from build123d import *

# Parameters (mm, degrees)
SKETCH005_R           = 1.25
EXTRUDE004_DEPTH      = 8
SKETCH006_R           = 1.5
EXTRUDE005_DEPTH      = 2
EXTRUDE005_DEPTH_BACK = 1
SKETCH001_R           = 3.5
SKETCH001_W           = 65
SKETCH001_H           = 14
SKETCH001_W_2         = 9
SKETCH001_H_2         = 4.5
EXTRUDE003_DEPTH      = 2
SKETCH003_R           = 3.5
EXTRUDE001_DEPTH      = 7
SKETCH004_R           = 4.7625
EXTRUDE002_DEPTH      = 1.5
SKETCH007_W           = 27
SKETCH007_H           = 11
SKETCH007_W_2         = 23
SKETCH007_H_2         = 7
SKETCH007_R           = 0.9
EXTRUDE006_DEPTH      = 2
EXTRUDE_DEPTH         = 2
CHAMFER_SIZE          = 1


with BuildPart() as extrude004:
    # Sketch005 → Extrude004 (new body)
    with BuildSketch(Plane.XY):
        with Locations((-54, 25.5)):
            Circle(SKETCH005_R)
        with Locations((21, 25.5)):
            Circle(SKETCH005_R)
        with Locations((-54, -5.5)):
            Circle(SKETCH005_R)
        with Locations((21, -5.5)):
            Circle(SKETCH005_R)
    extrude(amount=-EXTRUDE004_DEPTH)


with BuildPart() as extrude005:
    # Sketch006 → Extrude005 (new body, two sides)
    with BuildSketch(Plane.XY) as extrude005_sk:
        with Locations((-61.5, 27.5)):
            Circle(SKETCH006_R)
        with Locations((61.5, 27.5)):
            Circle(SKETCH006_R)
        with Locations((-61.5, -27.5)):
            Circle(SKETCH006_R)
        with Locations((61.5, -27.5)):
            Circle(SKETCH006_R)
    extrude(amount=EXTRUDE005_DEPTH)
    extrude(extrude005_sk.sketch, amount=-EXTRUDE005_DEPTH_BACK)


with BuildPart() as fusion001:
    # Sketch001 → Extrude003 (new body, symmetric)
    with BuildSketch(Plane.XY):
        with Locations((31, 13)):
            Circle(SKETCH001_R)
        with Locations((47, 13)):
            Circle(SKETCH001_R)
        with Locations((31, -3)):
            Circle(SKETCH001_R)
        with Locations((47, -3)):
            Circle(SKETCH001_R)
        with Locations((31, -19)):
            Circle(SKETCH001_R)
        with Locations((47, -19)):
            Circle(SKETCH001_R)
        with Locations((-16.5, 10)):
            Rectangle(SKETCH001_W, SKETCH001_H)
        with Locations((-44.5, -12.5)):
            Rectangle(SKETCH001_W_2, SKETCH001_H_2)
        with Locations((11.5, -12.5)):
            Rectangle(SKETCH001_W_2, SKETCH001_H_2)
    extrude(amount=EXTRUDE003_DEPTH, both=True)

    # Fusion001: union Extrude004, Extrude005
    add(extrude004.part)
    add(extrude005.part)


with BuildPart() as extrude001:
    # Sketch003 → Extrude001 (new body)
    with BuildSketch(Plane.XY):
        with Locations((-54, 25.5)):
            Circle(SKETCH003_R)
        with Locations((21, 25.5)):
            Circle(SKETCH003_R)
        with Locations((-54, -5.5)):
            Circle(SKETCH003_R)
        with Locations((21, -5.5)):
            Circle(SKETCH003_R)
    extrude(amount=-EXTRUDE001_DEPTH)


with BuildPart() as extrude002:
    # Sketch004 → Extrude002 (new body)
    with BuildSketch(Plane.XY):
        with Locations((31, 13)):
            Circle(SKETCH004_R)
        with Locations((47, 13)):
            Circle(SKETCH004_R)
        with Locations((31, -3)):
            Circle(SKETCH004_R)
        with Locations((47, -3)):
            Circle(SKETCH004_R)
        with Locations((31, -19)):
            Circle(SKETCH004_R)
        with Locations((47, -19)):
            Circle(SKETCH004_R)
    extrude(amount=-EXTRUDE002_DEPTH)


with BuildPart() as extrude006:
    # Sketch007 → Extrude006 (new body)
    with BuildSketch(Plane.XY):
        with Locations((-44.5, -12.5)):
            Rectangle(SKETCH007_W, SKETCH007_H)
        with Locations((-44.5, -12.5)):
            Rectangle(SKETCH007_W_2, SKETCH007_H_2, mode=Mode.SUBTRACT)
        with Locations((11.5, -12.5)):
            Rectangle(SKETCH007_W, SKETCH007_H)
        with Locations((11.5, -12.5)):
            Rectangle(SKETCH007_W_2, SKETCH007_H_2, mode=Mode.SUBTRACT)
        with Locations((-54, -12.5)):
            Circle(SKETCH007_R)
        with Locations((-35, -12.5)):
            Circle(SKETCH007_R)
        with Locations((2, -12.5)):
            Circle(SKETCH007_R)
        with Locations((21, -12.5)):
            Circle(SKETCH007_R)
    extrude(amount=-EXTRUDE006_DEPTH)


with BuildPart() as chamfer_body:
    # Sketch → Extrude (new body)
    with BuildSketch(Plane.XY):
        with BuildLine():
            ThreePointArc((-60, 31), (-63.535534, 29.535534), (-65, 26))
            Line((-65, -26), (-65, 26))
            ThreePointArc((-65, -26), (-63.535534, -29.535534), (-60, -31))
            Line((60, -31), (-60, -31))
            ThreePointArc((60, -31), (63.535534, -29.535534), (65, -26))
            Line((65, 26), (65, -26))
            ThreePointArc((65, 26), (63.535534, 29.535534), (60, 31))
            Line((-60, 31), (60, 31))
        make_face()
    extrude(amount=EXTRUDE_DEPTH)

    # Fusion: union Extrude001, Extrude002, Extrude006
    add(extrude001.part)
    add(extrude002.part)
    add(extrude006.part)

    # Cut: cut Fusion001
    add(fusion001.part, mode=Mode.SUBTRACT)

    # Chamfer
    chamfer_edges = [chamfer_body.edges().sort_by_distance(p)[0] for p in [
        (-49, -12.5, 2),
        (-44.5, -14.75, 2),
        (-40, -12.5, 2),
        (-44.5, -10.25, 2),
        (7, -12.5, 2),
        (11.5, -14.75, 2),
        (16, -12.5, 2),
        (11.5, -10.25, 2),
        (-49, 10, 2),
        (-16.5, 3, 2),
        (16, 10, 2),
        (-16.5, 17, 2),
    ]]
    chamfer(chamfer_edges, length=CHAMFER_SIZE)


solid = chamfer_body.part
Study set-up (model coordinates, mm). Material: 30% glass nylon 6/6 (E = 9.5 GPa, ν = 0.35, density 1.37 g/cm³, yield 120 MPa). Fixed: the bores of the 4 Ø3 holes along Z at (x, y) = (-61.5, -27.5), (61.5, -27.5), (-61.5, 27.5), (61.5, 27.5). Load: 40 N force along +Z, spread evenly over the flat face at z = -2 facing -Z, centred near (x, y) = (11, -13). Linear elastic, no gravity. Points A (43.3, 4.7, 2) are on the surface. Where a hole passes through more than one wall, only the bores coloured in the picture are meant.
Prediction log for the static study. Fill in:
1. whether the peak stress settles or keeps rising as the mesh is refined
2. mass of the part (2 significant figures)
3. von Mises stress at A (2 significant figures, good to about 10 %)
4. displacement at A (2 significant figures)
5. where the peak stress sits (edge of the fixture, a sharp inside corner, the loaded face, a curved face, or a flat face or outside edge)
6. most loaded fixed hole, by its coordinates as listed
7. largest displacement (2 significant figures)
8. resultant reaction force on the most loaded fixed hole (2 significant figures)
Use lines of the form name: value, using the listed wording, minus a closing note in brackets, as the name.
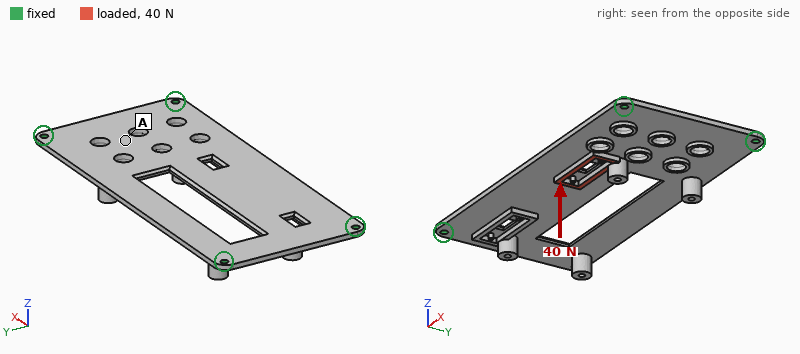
whether the peak stress settles or keeps rising as the mesh is refined: keeps rising
mass of the part: 21 g
von Mises stress at A: 4.8 MPa
displacement at A: 0.39 mm
where the peak stress sits: edge of the fixture
most loaded fixed hole, by its coordinates as listed: (61.5, -27.5)
largest displacement: 1.4 mm
resultant reaction force on the most loaded fixed hole: 20 N
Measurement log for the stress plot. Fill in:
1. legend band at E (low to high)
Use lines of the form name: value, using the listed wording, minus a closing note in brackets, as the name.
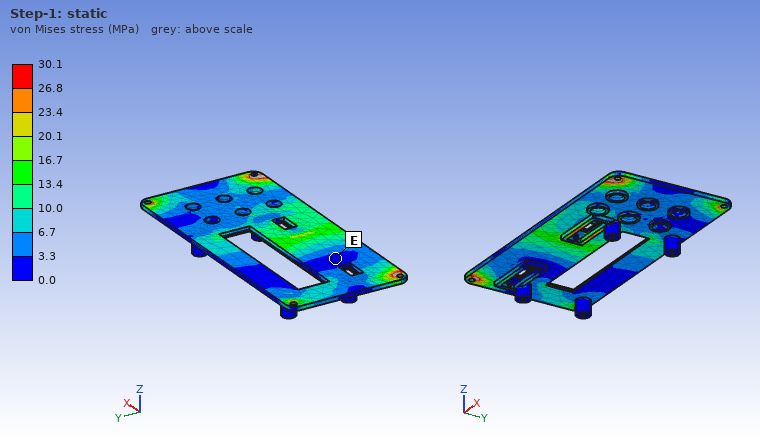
legend band at E: 0.0 to 3.3 MPa
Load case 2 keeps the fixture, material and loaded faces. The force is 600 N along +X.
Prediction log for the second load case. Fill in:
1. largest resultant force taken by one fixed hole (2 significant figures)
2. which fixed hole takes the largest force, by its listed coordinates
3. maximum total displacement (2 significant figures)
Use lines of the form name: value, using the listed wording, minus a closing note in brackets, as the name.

largest resultant force taken by one fixed hole: 270 N
which fixed hole takes the largest force, by its listed coordinates: (61.5, -27.5)
maximum total displacement: 1.1 mm
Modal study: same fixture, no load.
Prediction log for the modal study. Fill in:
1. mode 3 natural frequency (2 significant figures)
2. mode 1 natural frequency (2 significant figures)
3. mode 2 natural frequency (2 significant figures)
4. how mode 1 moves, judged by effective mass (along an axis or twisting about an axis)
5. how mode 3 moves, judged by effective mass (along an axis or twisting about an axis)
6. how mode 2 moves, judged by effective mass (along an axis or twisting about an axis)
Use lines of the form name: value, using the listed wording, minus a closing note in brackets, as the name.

mode 3 natural frequency: 870 Hz
mode 1 natural frequency: 320 Hz
mode 2 natural frequency: 520 Hz
how mode 1 moves, judged by effective mass: along Z
how mode 3 moves, judged by effective mass: twisting about Y
how mode 2 moves, judged by effective mass: twisting about X
